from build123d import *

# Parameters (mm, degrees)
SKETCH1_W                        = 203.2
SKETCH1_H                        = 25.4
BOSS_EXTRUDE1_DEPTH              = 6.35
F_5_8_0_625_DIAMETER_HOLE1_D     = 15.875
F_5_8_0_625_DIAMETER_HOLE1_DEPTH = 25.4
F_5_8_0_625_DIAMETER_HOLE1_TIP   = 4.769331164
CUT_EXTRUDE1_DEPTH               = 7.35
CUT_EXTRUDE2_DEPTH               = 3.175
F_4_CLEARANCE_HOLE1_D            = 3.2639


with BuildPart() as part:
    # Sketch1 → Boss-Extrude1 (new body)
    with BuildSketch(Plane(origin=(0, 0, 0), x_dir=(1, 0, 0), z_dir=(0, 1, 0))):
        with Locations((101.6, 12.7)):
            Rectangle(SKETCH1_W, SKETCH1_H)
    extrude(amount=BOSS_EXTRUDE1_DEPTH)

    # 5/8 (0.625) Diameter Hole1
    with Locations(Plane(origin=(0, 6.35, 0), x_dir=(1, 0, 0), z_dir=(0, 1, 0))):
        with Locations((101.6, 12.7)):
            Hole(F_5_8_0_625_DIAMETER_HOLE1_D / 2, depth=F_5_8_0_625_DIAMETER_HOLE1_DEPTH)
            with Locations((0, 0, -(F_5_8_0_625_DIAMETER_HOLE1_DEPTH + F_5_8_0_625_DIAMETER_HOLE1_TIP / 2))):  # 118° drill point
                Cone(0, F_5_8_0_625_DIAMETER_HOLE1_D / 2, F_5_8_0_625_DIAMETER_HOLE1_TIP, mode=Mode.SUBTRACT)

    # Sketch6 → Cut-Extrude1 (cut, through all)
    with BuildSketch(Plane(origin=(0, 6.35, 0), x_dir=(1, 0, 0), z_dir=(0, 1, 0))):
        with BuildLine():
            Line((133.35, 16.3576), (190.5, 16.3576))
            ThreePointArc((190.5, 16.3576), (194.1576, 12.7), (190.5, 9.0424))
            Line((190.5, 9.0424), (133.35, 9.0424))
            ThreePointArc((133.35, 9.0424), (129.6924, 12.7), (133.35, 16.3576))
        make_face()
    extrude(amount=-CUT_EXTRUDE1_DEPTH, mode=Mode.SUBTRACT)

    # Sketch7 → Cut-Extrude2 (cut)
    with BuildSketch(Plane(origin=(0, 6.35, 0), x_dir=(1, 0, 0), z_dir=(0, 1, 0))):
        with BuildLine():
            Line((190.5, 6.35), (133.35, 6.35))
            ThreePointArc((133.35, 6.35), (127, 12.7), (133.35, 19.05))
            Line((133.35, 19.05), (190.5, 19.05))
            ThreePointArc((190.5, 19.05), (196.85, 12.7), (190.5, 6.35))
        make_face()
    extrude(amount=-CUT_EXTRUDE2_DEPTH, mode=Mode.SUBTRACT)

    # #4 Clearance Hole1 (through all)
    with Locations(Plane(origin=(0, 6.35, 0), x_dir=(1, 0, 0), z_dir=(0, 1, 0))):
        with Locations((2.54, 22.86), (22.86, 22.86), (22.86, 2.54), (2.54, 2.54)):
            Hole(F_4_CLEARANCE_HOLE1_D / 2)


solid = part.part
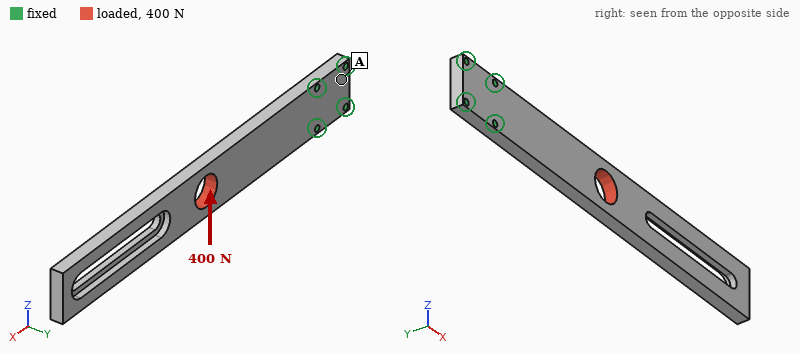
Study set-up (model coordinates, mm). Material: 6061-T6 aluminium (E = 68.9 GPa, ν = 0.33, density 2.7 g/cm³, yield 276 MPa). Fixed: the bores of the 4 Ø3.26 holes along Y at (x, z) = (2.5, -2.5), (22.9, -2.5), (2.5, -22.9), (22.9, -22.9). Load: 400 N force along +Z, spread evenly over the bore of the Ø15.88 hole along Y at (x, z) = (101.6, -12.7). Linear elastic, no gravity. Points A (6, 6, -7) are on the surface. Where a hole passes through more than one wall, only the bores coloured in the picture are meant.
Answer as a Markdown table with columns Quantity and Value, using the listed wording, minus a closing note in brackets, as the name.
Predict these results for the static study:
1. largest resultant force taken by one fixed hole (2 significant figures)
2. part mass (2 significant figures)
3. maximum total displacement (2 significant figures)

| Quantity | Value |
|---|---|
| largest resultant force taken by one fixed hole | 1.5 kN |
| part mass | 73 g |
| maximum total displacement | 0.33 mm |
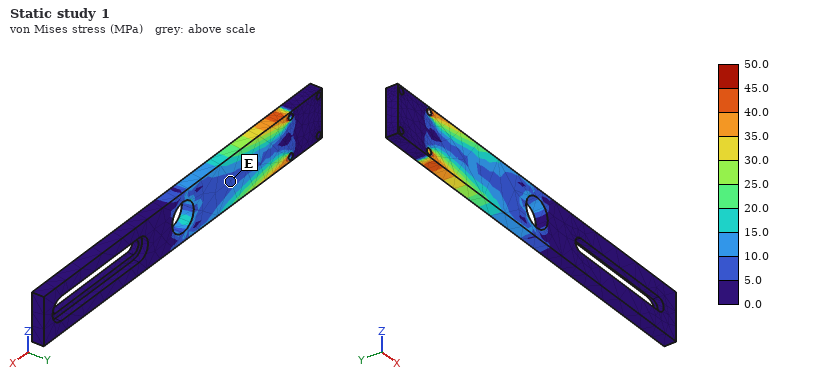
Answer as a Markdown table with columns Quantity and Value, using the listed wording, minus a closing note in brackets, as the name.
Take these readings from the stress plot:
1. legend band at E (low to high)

| Quantity | Value |
|---|---|
| legend band at E | 5.0 to 10.0 MPa |
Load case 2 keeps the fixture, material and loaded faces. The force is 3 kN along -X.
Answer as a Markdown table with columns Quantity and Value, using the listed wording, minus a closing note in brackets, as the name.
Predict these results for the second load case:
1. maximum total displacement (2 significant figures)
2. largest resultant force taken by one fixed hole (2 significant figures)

| Quantity | Value |
|---|---|
| maximum total displacement | 29 µm |
| largest resultant force taken by one fixed hole | 1.3 kN |
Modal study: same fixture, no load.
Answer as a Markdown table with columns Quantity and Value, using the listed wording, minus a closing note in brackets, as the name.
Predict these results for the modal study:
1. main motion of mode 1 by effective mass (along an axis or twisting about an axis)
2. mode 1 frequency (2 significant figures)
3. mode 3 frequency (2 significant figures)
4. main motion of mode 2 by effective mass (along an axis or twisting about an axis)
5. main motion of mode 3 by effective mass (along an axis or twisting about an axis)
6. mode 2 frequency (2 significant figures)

| Quantity | Value |
|---|---|
| main motion of mode 1 by effective mass | along Y |
| mode 1 frequency | 180 Hz |
| mode 3 frequency | 930 Hz |
| main motion of mode 2 by effective mass | along Z |
| main motion of mode 3 by effective mass | along Y |
| mode 2 frequency | 700 Hz |
